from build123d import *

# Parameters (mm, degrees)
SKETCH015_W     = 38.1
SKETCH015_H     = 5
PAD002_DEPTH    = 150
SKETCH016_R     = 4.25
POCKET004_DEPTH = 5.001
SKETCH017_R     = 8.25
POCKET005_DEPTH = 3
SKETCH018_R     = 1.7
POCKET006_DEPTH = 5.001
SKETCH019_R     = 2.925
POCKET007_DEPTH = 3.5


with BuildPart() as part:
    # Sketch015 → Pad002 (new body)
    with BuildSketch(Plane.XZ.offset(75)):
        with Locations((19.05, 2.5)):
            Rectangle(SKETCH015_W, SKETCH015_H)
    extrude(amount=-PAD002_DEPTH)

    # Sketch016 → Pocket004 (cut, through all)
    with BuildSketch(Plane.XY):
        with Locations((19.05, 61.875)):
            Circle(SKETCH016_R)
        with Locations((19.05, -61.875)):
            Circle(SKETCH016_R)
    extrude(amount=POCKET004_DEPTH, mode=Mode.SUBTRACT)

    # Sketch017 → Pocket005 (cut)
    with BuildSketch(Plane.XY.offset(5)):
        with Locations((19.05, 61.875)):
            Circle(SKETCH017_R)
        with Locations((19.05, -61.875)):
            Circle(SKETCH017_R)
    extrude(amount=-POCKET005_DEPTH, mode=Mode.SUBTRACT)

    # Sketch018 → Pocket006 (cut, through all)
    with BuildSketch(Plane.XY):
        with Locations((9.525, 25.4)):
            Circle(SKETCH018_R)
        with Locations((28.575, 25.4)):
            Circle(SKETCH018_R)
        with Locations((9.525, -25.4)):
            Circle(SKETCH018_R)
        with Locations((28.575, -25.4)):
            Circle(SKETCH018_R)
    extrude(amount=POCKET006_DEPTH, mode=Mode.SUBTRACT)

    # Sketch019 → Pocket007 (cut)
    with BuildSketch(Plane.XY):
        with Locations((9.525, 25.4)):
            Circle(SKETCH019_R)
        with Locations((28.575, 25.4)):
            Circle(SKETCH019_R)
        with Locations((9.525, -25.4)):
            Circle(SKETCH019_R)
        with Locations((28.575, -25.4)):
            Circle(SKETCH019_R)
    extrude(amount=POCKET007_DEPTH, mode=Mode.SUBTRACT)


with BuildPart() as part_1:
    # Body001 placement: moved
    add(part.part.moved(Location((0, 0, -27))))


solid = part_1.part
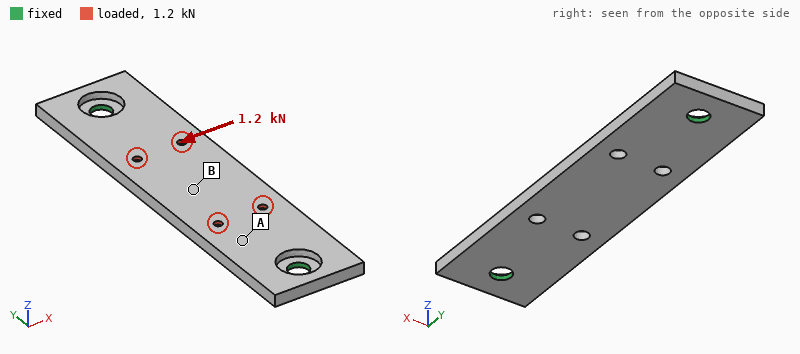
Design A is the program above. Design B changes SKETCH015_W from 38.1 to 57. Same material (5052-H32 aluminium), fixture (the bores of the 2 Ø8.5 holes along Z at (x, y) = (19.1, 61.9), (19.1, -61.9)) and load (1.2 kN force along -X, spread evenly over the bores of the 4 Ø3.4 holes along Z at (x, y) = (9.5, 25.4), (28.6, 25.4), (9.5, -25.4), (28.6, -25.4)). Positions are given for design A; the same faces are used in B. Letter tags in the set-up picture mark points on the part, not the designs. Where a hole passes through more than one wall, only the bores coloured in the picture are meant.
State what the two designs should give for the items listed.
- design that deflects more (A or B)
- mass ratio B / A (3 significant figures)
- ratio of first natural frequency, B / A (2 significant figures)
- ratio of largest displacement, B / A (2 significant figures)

A
1.53
0.91
0.59
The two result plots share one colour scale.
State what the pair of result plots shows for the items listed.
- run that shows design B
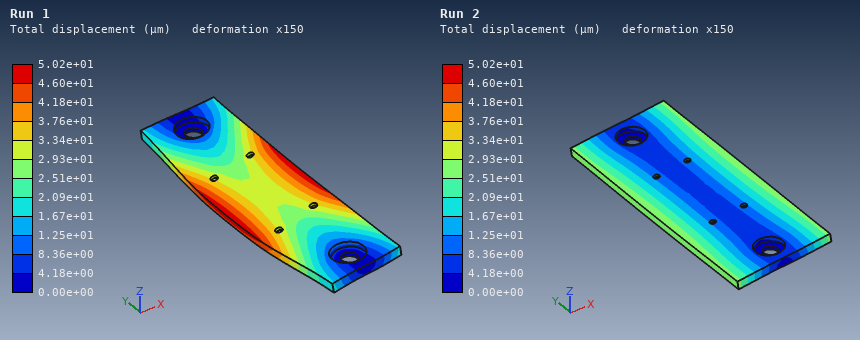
Run 2
